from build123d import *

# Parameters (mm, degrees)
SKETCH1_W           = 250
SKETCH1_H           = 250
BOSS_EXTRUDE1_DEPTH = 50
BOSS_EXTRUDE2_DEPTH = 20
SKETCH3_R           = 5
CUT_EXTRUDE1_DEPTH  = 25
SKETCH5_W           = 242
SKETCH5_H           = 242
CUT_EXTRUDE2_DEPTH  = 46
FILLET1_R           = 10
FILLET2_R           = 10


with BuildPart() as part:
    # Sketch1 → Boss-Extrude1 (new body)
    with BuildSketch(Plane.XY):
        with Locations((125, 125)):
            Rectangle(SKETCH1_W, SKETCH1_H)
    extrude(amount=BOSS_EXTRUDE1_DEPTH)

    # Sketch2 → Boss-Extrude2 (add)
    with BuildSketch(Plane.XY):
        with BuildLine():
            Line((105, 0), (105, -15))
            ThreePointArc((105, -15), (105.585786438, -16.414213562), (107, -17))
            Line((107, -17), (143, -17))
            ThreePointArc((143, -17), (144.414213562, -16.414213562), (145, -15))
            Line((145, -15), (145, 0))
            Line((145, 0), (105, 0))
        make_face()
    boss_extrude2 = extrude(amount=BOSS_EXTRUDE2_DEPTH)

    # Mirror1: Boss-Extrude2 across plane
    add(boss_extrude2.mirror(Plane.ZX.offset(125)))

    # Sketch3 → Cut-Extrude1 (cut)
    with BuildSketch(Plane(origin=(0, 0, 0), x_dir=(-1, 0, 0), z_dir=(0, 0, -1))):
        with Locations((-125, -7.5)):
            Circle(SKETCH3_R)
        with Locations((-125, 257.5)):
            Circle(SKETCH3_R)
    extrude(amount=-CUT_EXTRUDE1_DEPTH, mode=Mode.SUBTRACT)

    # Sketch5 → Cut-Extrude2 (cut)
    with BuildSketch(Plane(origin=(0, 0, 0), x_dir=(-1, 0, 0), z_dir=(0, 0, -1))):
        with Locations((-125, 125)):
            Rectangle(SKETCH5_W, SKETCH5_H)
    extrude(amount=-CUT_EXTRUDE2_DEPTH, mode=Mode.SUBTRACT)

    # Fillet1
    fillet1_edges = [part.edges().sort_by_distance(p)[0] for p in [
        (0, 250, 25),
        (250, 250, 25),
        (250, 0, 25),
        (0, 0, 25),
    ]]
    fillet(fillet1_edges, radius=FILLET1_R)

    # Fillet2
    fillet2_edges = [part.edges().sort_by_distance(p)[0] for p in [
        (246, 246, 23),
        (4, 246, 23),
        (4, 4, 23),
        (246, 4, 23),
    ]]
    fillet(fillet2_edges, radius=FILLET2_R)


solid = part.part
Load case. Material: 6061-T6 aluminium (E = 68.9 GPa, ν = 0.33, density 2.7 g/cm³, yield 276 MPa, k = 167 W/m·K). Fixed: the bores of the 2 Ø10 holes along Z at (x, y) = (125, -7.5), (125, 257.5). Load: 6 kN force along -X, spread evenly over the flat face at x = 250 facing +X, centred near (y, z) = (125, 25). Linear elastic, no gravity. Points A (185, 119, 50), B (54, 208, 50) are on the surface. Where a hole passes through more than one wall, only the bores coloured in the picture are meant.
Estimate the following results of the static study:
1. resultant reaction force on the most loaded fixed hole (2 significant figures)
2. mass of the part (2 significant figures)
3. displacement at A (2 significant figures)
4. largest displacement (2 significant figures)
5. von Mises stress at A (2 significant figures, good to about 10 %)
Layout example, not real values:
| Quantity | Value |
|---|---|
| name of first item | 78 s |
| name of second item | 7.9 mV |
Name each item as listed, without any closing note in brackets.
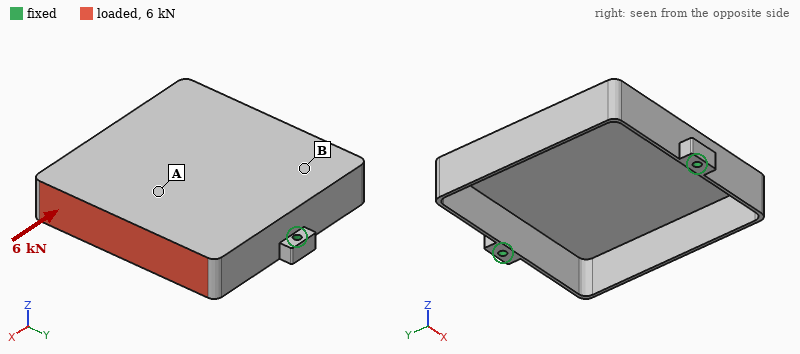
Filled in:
| Quantity | Value |
|---|---|
| resultant reaction force on the most loaded fixed hole | 3.0 kN |
| mass of the part | 1.2 kg |
| displacement at A | 0.73 mm |
| largest displacement | 2.1 mm |
| von Mises stress at A | 36 MPa |
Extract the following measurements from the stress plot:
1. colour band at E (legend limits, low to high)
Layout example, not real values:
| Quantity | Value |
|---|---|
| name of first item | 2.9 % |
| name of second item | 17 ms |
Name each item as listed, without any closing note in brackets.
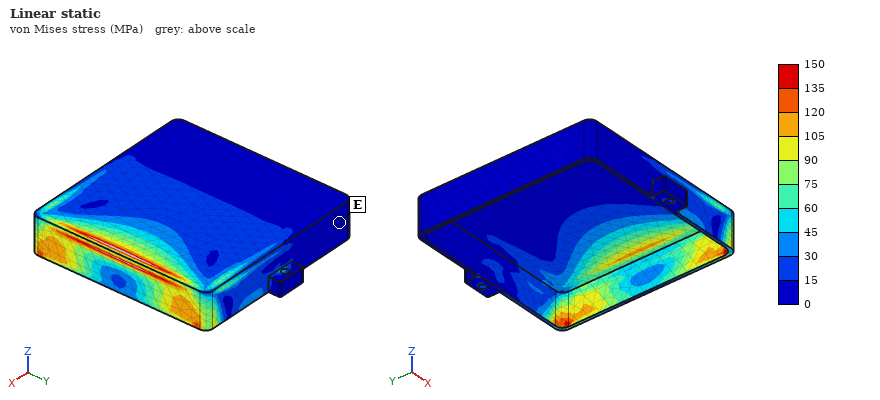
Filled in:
| Quantity | Value |
|---|---|
| colour band at E | 0 to 15 MPa |
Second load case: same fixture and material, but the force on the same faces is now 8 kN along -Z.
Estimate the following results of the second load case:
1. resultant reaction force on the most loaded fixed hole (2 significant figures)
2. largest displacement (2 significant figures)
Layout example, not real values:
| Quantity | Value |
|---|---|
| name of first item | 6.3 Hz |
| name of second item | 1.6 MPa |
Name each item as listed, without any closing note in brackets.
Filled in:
| Quantity | Value |
|---|---|
| resultant reaction force on the most loaded fixed hole | 4.0 kN |
| largest displacement | 1.7 mm |
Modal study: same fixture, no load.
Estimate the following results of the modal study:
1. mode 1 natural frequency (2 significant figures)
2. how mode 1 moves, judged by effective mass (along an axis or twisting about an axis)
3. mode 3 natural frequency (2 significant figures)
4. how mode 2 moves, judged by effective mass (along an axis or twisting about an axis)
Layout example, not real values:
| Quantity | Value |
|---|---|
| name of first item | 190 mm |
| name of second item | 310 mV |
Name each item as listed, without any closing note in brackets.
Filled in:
| Quantity | Value |
|---|---|
| mode 1 natural frequency | 450 Hz |
| how mode 1 moves, judged by effective mass | along Z |
| mode 3 natural frequency | 580 Hz |
| how mode 2 moves, judged by effective mass | along Y |
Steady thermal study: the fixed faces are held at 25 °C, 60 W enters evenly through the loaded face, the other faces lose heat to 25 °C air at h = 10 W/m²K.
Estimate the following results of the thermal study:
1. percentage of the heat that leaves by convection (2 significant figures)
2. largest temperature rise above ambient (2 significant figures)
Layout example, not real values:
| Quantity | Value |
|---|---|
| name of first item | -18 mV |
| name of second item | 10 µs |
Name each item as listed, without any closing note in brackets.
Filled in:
| Quantity | Value |
|---|---|
| percentage of the heat that leaves by convection | 49 % |
| largest temperature rise above ambient | 43 K |
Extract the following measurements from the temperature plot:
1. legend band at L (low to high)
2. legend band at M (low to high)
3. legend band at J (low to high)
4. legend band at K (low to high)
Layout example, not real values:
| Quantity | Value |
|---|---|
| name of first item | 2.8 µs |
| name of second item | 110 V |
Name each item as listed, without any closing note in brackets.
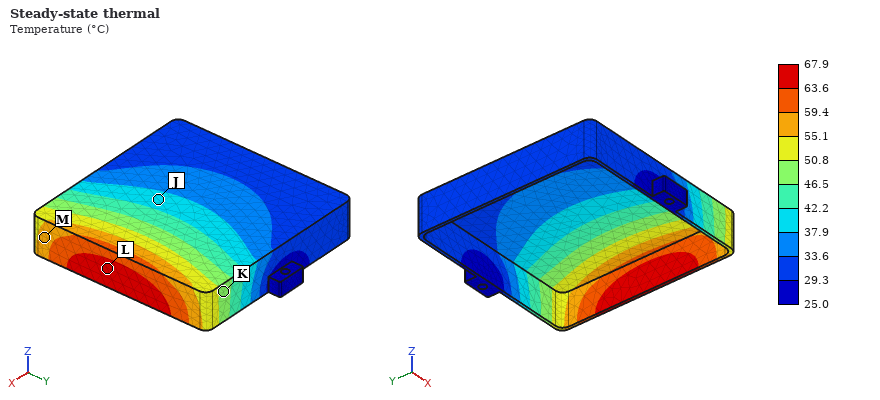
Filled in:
| Quantity | Value |
|---|---|
| legend band at L | 63.6 to 67.9 °C |
| legend band at M | 55.1 to 59.4 °C |
| legend band at J | 37.9 to 42.2 °C |
| legend band at K | 46.5 to 50.8 °C |
